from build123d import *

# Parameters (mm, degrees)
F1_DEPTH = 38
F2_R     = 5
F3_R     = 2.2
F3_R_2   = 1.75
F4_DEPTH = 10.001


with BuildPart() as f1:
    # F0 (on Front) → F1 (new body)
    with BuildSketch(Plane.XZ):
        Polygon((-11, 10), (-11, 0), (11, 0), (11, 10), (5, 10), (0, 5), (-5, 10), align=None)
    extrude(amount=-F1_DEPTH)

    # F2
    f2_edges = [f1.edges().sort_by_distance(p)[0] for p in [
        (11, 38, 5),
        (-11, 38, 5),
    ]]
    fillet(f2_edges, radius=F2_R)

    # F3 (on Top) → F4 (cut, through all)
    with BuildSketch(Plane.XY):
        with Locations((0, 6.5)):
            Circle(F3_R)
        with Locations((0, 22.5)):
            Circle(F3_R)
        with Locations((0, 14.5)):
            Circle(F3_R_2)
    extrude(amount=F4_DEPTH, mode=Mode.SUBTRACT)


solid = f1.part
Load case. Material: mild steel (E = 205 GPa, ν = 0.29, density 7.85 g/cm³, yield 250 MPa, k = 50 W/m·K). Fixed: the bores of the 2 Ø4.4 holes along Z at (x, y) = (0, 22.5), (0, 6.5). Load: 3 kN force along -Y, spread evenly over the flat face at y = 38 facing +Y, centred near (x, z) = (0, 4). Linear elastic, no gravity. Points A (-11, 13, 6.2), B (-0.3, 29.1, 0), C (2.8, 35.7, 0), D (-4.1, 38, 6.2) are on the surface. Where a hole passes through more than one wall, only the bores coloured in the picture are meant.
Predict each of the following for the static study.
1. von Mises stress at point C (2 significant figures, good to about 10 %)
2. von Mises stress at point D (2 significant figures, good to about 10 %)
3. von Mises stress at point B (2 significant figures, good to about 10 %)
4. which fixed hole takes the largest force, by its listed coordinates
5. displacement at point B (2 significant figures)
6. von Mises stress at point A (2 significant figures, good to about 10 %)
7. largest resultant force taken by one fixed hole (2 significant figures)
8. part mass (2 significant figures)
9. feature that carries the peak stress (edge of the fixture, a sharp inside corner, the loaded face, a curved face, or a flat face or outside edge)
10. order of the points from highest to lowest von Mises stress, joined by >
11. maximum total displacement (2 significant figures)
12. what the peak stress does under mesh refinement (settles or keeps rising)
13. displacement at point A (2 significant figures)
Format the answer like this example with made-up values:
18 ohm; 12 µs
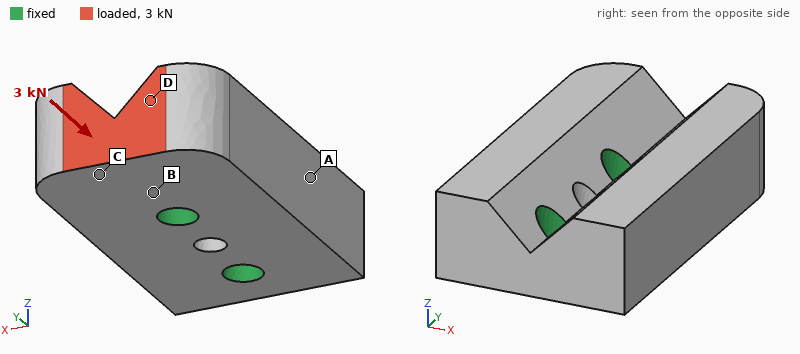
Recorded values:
31 MPa; 25 MPa; 38 MPa; (0, 22.5); 0.83 µm; 4.5 MPa; 2.4 kN; 55 g; edge of the fixture; B > C > D > A; 2.3 µm; keeps rising; 0.38 µm
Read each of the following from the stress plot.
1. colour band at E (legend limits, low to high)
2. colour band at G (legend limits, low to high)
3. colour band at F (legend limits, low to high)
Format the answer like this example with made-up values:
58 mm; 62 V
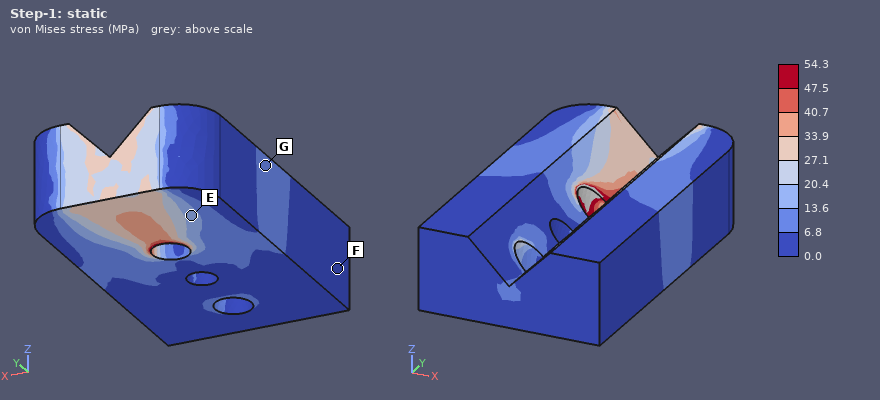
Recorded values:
13.6 to 20.4 MPa; 6.8 to 13.6 MPa; 0.0 to 6.8 MPa
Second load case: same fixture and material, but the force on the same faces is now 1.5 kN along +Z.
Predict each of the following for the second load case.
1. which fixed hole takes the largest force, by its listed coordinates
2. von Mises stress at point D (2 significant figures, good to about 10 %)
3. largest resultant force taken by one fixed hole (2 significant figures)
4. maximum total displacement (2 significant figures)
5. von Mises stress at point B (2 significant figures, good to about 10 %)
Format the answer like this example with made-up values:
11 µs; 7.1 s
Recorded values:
(0, 22.5); 38 MPa; 2.2 kN; 14 µm; 55 MPa
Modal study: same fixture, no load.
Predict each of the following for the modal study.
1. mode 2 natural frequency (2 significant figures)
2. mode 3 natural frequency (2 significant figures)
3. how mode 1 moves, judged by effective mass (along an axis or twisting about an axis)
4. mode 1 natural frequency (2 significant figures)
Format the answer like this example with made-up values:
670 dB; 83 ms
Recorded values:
23 kHz; 27 kHz; along Z; 21 kHz
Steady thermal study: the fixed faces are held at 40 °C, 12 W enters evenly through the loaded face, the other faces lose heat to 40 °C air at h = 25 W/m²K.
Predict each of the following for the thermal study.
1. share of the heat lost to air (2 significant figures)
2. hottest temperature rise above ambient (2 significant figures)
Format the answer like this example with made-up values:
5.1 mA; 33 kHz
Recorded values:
3.3 %; 27 K
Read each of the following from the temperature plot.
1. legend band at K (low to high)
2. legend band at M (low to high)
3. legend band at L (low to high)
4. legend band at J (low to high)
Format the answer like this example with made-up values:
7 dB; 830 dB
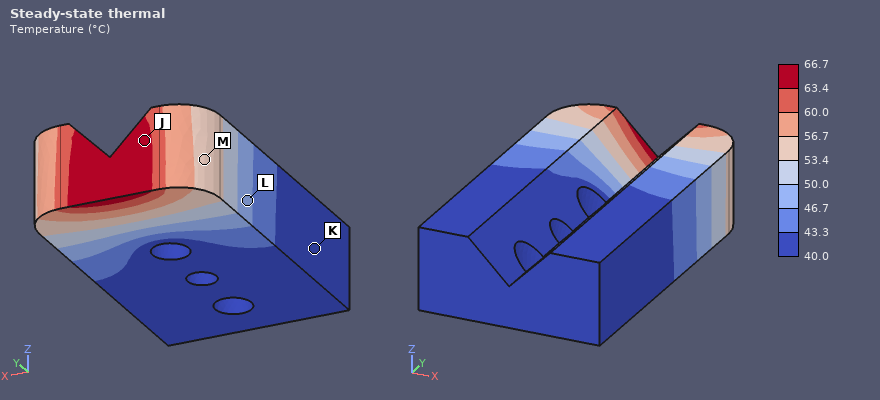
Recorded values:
40.0 to 43.3 °C; 53.4 to 56.7 °C; 46.7 to 50.0 °C; 63.4 to 66.7 °C
